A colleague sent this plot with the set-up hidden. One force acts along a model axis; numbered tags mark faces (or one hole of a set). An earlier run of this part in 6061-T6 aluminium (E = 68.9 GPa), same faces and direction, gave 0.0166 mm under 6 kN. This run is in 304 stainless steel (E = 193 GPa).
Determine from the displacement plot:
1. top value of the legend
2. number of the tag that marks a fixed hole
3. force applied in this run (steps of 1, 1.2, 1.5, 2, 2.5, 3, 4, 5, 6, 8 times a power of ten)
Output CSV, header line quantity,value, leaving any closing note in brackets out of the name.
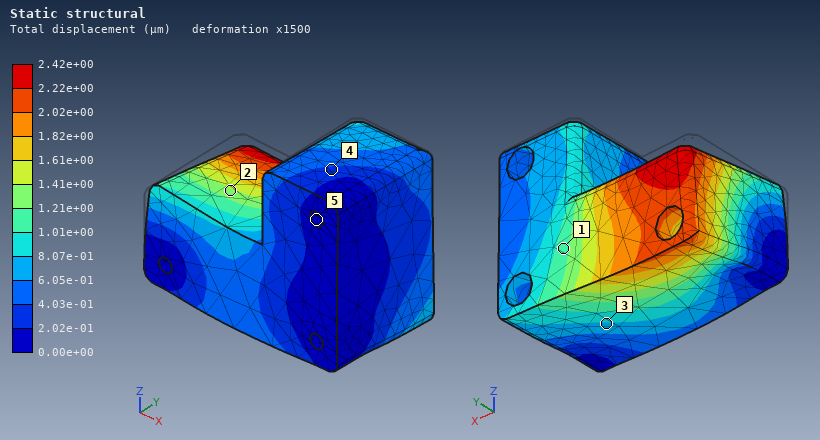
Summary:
quantity,value
top value of the legend,2.42e+00 µm
number of the tag that marks a fixed hole,5
force applied in this run,2.5 kN
